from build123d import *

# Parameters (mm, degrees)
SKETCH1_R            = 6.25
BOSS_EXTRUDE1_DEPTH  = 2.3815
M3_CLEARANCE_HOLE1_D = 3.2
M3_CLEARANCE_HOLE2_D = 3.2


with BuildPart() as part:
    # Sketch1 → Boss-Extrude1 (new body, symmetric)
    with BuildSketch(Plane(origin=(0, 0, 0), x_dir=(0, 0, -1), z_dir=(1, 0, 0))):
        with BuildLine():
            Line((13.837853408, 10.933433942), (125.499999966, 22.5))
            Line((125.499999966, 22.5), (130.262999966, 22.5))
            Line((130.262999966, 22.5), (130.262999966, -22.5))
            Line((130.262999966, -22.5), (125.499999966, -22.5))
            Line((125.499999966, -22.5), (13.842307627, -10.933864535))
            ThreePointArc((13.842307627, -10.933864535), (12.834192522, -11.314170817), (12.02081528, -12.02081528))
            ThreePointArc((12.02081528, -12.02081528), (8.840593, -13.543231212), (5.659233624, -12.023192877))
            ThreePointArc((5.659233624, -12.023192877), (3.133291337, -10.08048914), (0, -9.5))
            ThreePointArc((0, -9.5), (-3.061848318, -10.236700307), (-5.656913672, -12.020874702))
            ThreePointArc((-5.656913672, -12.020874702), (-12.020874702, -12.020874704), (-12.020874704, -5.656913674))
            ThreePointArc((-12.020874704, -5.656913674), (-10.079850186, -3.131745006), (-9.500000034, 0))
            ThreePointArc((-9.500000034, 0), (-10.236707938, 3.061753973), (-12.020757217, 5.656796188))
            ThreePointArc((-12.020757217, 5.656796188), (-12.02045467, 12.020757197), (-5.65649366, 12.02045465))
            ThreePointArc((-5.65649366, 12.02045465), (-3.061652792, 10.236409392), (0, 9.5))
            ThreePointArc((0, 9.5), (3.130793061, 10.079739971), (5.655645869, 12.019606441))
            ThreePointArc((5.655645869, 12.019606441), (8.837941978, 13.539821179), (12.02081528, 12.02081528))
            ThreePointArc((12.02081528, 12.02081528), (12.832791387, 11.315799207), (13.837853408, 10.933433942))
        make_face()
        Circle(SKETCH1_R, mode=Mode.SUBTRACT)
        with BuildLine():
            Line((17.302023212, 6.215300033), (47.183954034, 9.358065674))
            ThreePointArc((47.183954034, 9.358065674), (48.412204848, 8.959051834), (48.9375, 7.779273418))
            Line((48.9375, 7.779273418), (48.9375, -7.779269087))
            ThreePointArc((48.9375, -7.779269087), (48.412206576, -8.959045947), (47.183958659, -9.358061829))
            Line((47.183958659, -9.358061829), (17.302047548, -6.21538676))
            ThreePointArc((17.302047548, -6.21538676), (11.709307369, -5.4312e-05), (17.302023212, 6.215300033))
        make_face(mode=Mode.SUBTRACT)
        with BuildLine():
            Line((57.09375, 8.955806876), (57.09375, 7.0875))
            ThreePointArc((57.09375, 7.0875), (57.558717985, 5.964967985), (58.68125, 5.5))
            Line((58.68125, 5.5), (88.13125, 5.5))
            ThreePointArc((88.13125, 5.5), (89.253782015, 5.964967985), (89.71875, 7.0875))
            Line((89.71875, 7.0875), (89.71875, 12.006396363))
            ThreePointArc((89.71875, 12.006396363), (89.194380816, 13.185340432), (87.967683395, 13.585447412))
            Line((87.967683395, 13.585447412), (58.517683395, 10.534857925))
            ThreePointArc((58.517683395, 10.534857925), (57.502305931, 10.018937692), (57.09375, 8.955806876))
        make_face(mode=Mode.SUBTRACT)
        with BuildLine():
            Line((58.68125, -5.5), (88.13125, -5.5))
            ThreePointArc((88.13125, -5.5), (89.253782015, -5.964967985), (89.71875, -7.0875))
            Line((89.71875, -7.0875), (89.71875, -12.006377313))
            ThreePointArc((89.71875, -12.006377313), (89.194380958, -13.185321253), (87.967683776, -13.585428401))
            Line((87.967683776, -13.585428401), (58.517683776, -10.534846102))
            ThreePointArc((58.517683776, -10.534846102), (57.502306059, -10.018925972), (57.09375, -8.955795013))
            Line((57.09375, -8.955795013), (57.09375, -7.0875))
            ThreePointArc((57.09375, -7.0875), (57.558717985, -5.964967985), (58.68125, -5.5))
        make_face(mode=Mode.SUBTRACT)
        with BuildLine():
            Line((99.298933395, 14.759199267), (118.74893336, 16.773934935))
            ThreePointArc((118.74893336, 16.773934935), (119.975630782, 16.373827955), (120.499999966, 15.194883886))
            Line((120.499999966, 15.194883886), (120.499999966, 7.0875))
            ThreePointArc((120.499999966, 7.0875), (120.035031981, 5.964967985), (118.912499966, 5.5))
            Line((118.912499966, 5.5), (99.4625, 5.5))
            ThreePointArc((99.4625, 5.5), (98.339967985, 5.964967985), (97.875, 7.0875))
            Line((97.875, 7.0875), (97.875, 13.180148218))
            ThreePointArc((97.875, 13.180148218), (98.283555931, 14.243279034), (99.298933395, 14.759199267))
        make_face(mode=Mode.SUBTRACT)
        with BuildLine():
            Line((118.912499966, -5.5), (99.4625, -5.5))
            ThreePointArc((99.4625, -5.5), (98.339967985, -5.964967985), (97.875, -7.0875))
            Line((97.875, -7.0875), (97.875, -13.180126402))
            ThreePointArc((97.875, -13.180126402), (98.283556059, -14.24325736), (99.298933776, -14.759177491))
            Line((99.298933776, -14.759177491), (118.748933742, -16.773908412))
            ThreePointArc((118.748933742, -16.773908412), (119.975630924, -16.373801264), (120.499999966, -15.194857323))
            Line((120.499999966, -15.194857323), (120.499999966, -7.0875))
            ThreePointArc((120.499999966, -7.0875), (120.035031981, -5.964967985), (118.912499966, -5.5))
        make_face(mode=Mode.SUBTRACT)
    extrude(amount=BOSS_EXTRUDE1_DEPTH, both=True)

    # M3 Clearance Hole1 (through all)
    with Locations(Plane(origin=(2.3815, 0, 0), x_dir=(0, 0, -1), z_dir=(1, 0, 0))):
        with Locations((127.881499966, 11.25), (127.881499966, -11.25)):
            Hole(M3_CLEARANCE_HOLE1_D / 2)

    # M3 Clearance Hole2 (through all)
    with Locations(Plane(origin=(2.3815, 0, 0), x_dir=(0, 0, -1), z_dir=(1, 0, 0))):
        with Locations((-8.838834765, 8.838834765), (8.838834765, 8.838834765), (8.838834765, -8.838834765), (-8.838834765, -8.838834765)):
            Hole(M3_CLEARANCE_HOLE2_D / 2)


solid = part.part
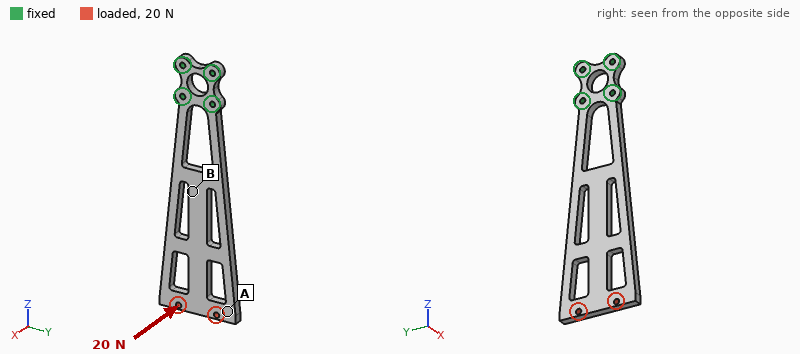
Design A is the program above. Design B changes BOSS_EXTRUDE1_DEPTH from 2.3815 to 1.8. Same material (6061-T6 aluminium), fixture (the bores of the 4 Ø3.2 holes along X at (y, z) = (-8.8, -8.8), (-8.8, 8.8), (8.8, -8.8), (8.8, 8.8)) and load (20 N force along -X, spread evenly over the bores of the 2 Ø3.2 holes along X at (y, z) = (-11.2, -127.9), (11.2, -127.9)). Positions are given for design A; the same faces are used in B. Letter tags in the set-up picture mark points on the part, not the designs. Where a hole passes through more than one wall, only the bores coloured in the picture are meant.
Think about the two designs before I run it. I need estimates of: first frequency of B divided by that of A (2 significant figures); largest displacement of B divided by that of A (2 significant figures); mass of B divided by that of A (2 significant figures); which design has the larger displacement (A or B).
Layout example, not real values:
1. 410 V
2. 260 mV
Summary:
1. 0.76
2. 2.3
3. 0.76
4. B
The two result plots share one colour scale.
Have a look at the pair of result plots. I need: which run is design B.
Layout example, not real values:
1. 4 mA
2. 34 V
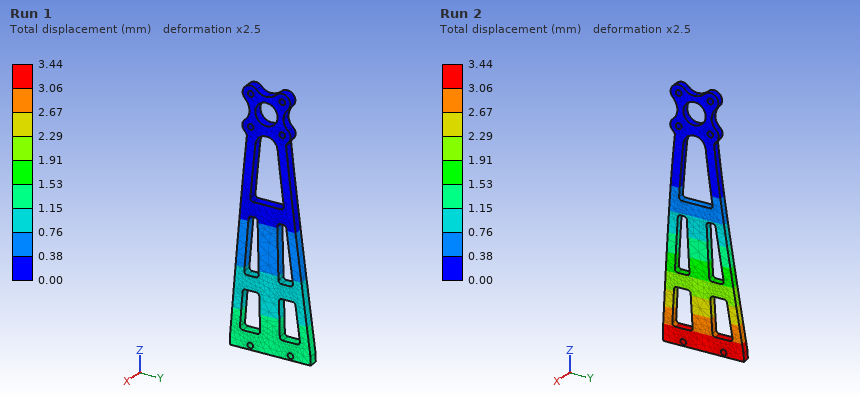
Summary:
1. Run 2
